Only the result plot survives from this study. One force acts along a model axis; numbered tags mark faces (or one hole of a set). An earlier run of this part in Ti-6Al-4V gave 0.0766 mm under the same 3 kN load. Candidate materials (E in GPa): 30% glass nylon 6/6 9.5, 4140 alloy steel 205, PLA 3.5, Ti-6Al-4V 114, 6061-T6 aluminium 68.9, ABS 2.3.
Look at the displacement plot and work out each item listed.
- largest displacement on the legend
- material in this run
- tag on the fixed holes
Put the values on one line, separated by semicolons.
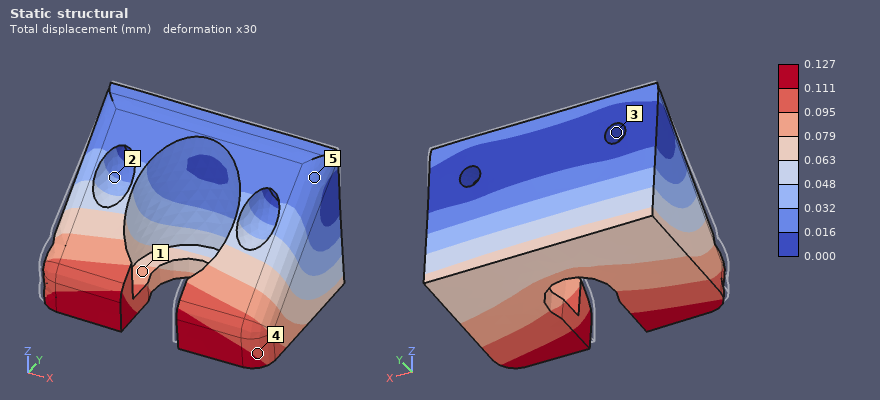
0.127 mm; 6061-T6 aluminium; 3
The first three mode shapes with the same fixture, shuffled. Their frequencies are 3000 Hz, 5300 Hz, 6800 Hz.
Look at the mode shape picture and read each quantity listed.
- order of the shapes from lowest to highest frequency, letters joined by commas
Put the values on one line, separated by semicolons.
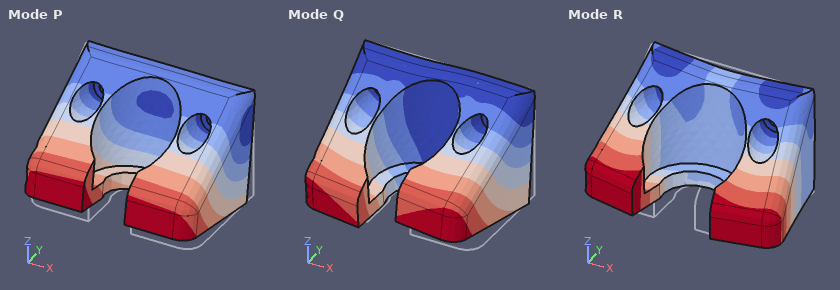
P, Q, R
